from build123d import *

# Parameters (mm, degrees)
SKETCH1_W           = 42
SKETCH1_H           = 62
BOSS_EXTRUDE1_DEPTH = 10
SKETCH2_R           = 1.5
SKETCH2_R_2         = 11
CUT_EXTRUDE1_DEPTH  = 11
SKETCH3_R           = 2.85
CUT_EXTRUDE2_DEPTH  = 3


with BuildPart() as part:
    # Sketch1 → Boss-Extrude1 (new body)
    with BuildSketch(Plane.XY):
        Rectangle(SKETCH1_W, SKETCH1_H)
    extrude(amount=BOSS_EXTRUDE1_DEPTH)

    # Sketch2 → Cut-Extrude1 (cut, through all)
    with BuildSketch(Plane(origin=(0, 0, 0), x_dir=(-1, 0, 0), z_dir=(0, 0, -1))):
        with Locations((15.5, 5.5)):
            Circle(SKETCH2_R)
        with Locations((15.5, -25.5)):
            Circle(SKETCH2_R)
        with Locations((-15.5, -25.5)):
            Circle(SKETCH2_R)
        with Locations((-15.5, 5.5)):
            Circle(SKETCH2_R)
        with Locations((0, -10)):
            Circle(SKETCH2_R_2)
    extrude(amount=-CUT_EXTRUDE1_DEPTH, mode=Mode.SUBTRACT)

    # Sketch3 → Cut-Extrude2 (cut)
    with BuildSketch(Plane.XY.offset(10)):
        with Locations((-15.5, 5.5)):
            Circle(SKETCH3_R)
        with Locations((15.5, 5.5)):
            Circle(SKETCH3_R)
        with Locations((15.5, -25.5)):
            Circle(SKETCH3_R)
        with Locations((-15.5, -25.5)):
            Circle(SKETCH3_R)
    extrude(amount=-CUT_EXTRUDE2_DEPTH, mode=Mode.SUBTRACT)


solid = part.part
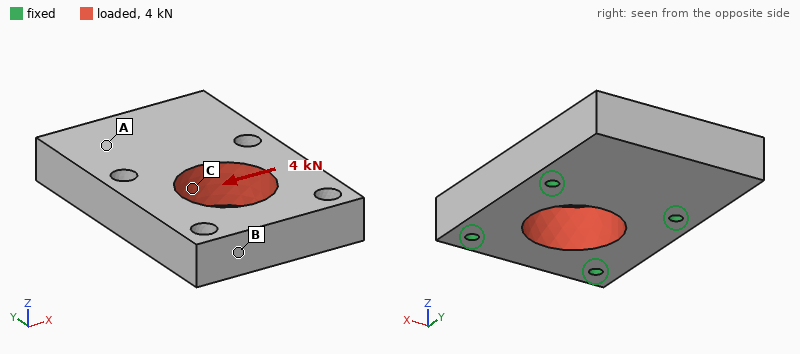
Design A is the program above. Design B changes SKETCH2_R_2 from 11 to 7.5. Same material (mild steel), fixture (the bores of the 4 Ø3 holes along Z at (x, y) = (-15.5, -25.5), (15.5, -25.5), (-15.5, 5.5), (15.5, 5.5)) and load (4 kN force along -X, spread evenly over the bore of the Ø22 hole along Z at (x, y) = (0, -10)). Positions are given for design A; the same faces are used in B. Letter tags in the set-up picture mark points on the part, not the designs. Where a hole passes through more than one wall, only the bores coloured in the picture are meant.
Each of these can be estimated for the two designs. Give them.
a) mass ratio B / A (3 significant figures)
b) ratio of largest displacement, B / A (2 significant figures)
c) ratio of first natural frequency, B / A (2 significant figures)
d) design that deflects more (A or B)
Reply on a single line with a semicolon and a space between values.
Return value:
1.09; 0.91; 1.0; A
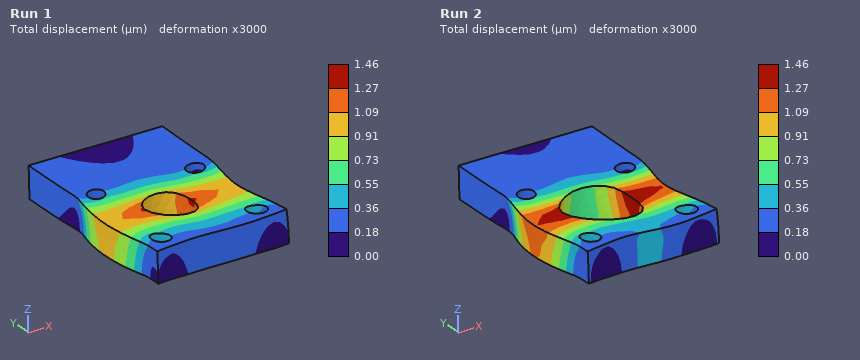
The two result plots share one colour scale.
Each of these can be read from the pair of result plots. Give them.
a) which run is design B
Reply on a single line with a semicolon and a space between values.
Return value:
Run 1
